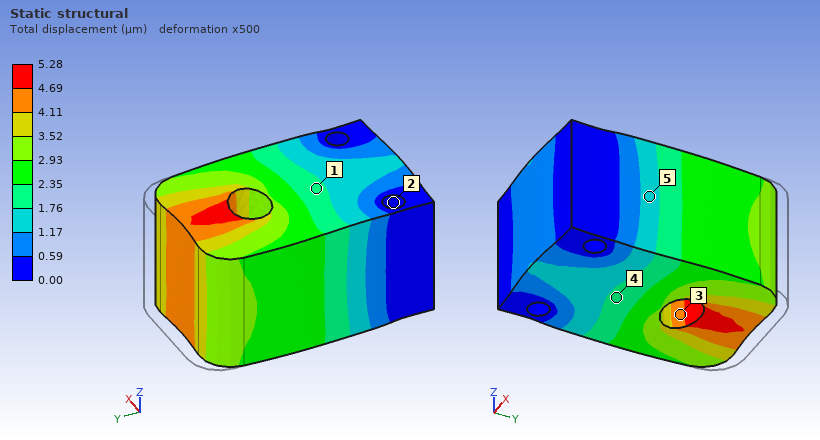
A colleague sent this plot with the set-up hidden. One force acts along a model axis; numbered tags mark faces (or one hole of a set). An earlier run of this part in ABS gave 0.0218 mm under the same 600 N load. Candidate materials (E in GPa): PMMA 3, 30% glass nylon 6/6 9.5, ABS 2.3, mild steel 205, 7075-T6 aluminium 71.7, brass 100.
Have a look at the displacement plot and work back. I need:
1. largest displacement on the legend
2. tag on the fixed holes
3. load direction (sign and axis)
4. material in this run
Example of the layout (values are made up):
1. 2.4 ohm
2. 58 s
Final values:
1. 5.28 µm
2. 2
3. -Y
4. 30% glass nylon 6/6
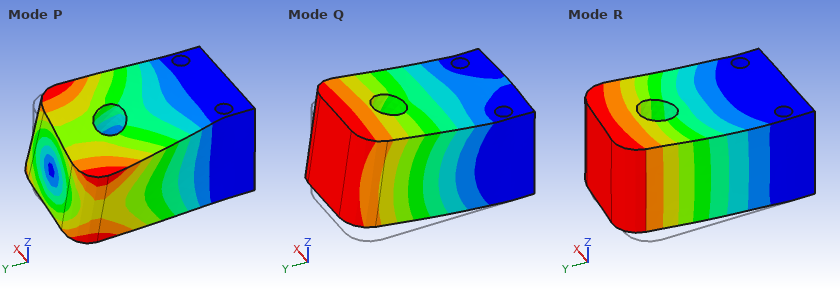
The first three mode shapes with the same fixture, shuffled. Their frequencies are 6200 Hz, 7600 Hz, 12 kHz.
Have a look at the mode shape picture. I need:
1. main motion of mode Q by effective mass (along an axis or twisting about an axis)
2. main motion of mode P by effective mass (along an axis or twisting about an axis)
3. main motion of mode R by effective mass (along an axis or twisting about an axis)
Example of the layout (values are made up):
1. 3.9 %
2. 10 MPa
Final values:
1. along Z
2. twisting about Y
3. along X
